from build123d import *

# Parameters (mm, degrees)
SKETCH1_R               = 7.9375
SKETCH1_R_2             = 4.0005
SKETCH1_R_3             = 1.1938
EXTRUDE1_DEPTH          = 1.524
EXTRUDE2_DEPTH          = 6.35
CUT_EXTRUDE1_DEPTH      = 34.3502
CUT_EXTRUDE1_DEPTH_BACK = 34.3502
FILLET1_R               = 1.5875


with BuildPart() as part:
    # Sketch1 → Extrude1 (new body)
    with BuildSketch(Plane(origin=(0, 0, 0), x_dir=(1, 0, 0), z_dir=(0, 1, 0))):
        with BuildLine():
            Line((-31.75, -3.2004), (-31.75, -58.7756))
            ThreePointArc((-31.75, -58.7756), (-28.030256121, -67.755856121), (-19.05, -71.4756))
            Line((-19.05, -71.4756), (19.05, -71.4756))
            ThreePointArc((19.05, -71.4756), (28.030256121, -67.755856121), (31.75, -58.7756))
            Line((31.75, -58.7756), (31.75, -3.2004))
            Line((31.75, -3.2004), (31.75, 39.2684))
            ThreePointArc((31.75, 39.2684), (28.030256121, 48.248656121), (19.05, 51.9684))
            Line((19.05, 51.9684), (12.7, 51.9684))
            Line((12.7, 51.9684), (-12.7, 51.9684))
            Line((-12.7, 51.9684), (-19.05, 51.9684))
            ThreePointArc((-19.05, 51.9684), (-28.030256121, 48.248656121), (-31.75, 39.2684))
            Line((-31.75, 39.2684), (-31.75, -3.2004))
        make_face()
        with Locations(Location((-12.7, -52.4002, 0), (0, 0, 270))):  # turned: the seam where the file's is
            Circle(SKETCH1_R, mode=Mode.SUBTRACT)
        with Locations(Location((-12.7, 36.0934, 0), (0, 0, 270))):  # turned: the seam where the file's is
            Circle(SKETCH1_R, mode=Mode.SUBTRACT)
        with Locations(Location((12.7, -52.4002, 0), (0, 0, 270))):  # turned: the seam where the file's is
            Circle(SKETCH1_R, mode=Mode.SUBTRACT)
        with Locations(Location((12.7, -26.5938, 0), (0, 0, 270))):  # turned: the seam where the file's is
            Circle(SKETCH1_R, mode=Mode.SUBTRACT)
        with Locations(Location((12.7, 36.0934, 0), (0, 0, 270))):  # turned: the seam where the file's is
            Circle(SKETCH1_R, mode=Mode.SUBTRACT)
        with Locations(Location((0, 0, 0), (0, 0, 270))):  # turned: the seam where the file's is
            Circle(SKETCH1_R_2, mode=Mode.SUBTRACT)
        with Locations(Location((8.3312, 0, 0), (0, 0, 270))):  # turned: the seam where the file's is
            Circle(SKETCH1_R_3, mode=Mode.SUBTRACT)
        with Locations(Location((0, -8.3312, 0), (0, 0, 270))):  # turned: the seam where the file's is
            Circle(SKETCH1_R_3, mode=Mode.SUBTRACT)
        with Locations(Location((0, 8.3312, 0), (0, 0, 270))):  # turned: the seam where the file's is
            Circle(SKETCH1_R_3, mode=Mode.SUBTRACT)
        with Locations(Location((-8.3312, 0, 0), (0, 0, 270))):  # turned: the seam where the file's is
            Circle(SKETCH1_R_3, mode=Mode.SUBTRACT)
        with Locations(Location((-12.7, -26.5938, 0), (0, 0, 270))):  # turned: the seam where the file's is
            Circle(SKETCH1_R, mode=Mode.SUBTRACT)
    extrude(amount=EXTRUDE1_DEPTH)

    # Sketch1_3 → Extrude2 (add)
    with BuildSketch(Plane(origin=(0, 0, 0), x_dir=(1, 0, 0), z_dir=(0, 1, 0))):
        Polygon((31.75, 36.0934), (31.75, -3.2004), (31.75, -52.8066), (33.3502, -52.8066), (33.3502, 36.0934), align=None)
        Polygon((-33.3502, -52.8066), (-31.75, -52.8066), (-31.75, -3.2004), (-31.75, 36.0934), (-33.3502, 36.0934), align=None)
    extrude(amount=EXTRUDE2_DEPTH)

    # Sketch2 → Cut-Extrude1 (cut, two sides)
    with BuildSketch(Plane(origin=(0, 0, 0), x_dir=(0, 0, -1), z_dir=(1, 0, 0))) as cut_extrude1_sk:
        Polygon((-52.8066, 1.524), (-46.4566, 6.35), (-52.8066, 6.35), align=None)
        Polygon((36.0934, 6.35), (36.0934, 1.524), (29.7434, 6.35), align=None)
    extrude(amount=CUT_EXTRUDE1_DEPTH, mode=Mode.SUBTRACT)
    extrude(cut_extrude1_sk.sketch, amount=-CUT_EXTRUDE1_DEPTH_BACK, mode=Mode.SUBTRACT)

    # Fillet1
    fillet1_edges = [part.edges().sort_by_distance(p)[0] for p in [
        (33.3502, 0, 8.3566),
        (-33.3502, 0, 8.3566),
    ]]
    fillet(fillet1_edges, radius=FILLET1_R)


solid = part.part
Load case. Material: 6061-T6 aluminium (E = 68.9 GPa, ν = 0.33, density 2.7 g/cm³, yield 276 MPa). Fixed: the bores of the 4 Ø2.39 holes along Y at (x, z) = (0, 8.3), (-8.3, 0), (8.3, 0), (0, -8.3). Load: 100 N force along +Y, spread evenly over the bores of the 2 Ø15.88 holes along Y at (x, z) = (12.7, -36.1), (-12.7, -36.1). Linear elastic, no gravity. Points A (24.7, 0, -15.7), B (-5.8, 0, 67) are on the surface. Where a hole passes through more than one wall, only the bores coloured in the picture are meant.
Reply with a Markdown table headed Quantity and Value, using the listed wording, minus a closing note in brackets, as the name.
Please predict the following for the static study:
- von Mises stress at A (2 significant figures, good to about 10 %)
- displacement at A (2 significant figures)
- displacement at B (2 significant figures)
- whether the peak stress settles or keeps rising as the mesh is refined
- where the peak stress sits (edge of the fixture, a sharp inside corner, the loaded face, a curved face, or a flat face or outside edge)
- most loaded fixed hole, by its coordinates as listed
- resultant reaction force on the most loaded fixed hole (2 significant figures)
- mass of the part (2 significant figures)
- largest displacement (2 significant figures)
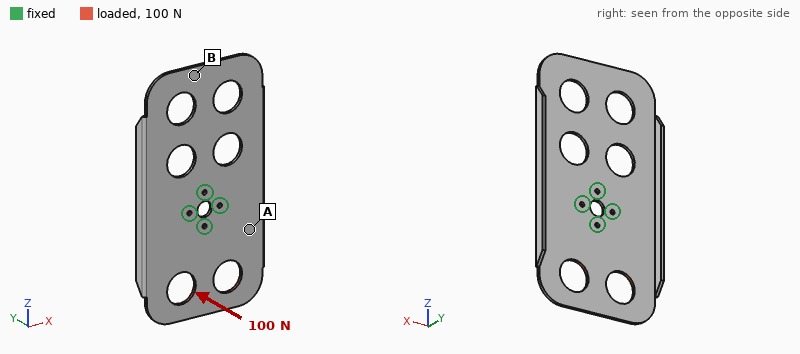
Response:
| Quantity | Value |
|---|---|
| von Mises stress at A | 24 MPa |
| displacement at A | 0.22 mm |
| displacement at B | 0.58 mm |
| whether the peak stress settles or keeps rising as the mesh is refined | keeps rising |
| where the peak stress sits | edge of the fixture |
| most loaded fixed hole, by its coordinates as listed | (0, -8.3) |
| resultant reaction force on the most loaded fixed hole | 150 N |
| mass of the part | 31 g |
| largest displacement | 1.00 mm |
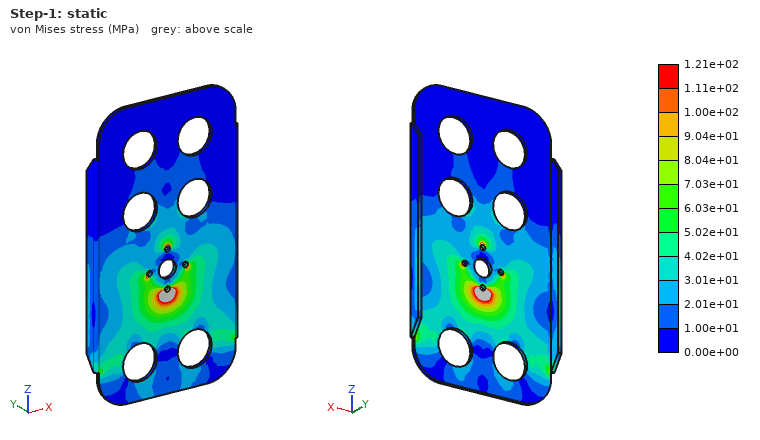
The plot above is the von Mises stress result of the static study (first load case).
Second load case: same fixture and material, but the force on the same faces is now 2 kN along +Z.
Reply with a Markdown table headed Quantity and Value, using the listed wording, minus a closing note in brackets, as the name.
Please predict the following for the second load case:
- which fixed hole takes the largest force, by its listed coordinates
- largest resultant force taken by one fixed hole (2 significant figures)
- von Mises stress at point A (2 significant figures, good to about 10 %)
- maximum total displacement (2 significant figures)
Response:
| Quantity | Value |
|---|---|
| which fixed hole takes the largest force, by its listed coordinates | (0, -8.3) |
| largest resultant force taken by one fixed hole | 660 N |
| von Mises stress at point A | 14 MPa |
| maximum total displacement | 46 µm |
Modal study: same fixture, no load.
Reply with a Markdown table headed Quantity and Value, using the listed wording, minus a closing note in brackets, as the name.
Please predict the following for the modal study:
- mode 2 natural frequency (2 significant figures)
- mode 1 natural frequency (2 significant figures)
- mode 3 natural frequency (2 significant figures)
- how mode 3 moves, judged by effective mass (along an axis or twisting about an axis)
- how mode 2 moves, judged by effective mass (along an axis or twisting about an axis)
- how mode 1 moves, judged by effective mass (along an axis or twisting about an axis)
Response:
| Quantity | Value |
|---|---|
| mode 2 natural frequency | 590 Hz |
| mode 1 natural frequency | 380 Hz |
| mode 3 natural frequency | 830 Hz |
| how mode 3 moves, judged by effective mass | along Y |
| how mode 2 moves, judged by effective mass | twisting about Z |
| how mode 1 moves, judged by effective mass | along Y |
